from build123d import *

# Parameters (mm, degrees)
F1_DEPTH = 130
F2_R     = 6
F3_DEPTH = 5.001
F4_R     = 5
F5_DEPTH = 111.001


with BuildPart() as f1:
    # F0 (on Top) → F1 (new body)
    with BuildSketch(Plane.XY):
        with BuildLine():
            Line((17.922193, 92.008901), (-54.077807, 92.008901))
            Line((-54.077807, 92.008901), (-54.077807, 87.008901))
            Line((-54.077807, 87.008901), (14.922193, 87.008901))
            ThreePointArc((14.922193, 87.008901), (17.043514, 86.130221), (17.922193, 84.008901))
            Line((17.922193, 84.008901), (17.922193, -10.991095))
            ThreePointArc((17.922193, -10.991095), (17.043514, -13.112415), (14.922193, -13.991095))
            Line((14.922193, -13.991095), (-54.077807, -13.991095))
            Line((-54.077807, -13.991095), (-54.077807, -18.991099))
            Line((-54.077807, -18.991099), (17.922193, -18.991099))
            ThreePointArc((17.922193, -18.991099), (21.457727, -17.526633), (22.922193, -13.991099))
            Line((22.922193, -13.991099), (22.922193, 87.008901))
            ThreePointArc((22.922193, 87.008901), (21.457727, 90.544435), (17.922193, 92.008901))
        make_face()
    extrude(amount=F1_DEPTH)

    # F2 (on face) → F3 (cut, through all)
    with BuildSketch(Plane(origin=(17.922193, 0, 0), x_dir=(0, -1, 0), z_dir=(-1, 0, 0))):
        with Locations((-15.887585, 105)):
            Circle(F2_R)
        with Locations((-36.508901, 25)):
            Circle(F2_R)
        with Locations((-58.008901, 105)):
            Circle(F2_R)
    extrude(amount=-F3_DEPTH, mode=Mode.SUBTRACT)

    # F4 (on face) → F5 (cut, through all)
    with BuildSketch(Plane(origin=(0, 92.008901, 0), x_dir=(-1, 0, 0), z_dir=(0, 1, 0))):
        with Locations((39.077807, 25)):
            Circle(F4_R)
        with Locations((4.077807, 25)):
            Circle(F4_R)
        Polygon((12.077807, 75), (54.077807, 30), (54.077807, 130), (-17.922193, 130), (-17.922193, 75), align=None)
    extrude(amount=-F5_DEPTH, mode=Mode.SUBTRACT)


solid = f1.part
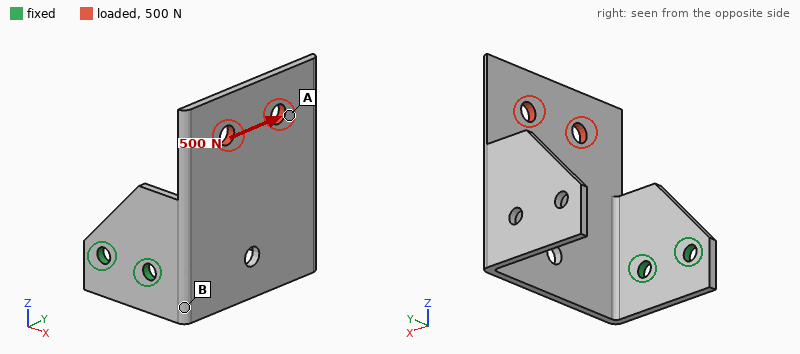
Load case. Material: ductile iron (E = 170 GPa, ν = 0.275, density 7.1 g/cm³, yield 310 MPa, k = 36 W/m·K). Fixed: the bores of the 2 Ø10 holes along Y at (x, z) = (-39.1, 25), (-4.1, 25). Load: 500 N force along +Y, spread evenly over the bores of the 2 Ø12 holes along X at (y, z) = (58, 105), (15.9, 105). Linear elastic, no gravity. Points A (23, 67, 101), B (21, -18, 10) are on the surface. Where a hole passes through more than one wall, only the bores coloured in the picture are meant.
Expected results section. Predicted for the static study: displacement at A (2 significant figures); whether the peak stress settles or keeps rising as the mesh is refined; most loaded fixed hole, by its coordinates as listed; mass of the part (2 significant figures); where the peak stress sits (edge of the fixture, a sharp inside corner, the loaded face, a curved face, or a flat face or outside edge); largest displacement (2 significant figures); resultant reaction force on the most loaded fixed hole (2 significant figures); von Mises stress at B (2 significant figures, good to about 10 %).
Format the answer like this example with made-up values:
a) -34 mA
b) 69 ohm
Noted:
a) 0.54 mm
b) keeps rising
c) (-4.1, 25)
d) 800 g
e) edge of the fixture
f) 0.72 mm
g) 630 N
h) 48 MPa
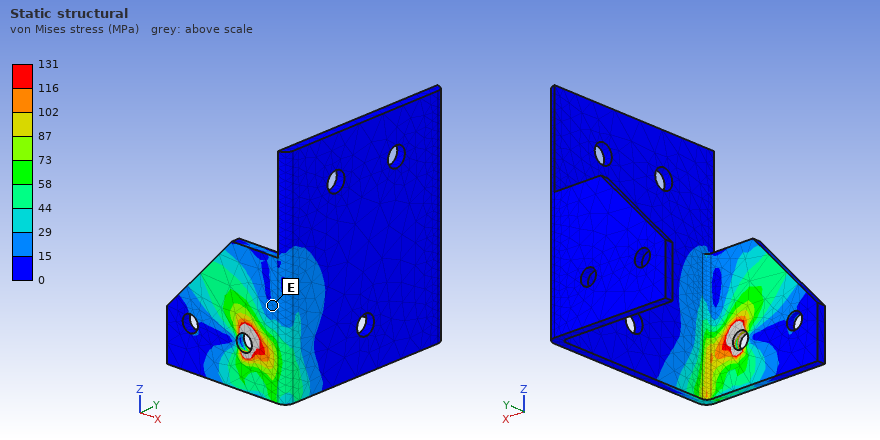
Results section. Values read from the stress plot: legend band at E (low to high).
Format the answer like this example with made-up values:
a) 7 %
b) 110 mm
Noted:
a) 15 to 29 MPa
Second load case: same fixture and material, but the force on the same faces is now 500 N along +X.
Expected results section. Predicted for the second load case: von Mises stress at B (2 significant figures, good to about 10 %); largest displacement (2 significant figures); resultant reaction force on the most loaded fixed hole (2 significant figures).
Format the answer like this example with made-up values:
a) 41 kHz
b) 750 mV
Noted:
a) 39 MPa
b) 1.6 mm
c) 990 N
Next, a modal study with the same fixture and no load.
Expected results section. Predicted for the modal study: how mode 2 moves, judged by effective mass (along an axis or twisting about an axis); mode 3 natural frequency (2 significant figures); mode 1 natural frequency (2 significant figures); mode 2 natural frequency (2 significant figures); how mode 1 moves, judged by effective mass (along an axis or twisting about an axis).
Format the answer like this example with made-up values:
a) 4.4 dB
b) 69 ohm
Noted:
a) along Z
b) 380 Hz
c) 130 Hz
d) 210 Hz
e) along X
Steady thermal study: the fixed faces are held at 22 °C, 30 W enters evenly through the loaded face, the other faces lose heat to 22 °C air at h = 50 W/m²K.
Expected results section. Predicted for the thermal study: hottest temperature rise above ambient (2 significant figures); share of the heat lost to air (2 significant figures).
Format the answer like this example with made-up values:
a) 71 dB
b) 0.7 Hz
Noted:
a) 51 K
b) 95 %
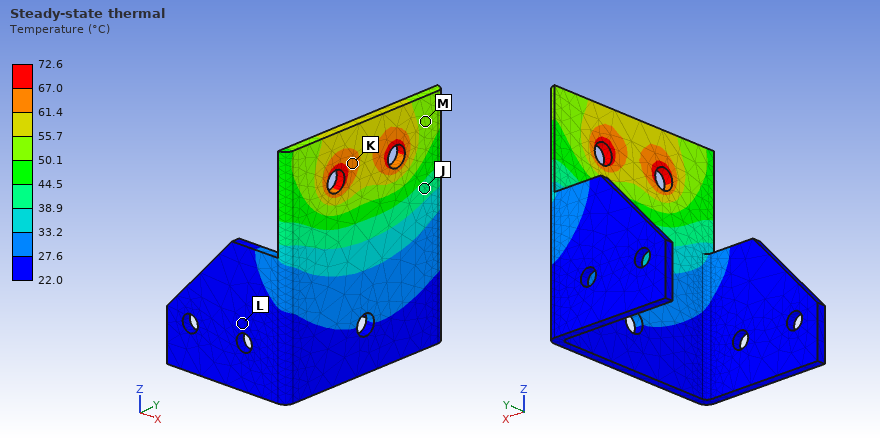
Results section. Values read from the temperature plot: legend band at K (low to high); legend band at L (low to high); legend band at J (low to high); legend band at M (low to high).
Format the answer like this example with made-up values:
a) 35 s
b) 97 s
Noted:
a) 61.4 to 67.0 °C
b) 22.0 to 27.6 °C
c) 38.9 to 44.5 °C
d) 50.1 to 55.7 °C
